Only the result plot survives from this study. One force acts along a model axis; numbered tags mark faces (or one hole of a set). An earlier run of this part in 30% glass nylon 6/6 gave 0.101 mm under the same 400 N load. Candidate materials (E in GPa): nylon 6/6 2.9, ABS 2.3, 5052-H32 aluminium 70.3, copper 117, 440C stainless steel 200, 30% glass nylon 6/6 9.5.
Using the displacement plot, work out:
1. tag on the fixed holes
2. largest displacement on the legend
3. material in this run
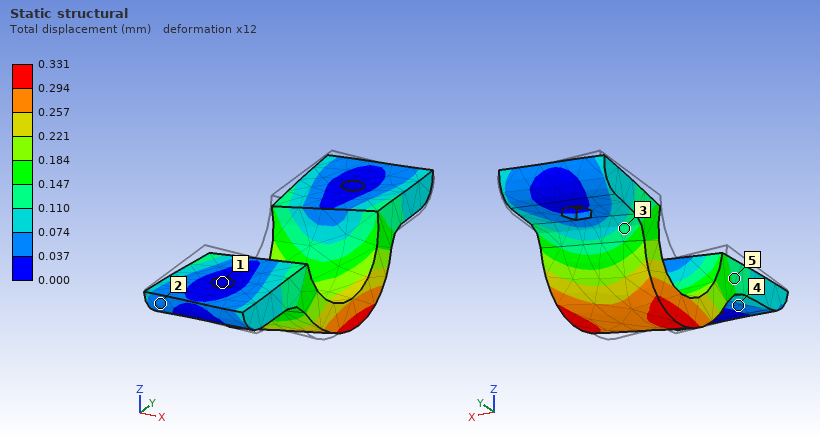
1
0.331 mm
nylon 6/6
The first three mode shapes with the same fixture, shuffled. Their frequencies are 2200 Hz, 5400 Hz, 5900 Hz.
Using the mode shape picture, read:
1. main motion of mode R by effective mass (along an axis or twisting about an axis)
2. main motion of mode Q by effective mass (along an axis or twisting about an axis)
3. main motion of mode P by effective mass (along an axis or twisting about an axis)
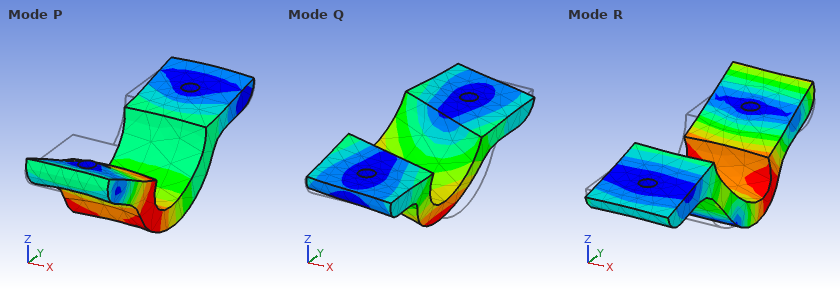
along Y
along X
along Z
